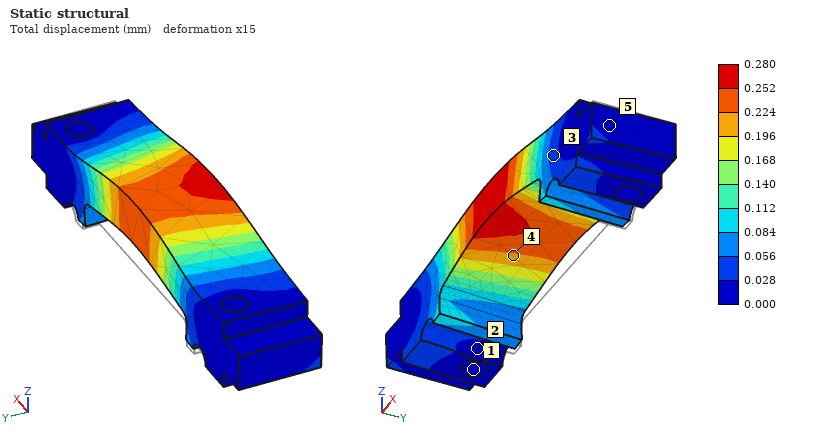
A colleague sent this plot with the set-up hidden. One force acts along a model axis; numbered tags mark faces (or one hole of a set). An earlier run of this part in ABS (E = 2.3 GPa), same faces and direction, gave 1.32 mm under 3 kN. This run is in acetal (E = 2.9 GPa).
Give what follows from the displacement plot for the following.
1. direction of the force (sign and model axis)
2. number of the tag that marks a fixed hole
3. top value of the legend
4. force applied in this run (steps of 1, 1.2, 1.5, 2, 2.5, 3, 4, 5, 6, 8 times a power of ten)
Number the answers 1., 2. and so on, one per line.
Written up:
1. +Z
2. 1
3. 0.280 mm
4. 800 N
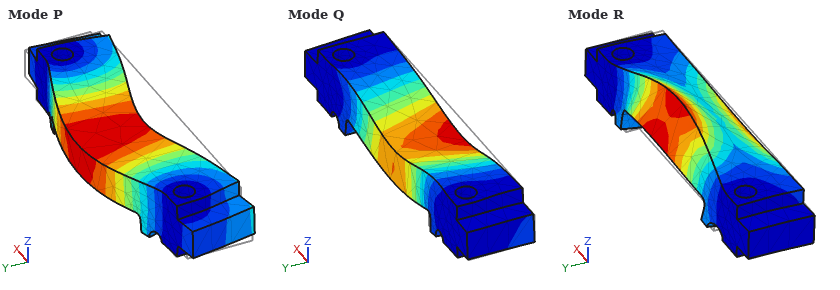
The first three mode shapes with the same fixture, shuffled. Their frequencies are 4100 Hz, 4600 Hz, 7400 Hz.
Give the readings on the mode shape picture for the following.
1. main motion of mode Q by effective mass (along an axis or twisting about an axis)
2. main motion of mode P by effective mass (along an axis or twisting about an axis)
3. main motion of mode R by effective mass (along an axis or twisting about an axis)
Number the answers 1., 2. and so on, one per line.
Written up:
1. along Z
2. along Y
3. twisting about X
